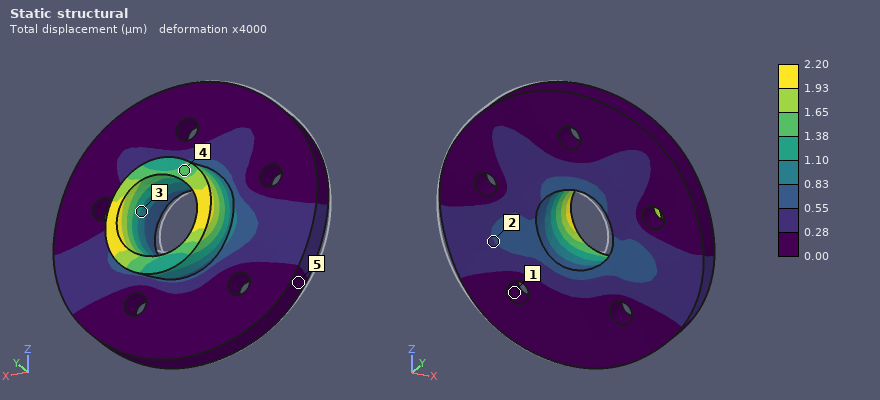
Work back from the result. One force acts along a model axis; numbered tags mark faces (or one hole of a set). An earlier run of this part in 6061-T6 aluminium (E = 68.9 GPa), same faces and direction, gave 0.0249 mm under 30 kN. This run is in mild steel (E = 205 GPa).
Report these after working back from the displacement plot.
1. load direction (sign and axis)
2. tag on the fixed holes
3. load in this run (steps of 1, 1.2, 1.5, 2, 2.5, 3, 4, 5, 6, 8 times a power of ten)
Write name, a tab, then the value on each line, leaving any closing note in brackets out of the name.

load direction	+X
tag on the fixed holes	1
load in this run	8 kN
